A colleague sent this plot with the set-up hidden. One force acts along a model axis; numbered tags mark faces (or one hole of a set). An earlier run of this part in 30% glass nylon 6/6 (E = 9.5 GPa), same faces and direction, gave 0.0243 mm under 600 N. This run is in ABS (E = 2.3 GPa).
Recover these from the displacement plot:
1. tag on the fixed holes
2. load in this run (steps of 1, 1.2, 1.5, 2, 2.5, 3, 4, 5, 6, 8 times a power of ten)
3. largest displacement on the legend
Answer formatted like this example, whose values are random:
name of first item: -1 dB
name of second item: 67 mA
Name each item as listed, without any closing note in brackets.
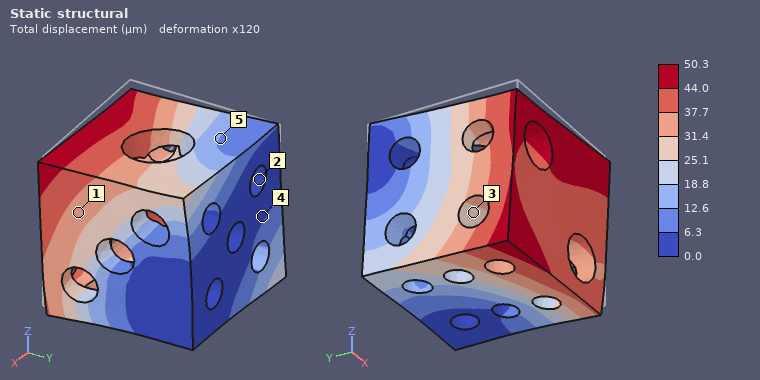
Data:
tag on the fixed holes: 2
load in this run: 300 N
largest displacement on the legend: 50.3 µm
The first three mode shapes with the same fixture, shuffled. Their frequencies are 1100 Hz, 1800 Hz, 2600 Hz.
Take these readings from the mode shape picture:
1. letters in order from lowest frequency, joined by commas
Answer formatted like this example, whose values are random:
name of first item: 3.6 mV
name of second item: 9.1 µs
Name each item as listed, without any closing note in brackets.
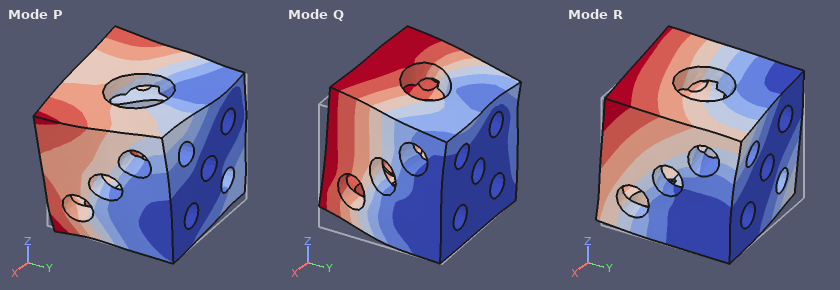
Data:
letters in order from lowest frequency, joined by commas: R, Q, P
